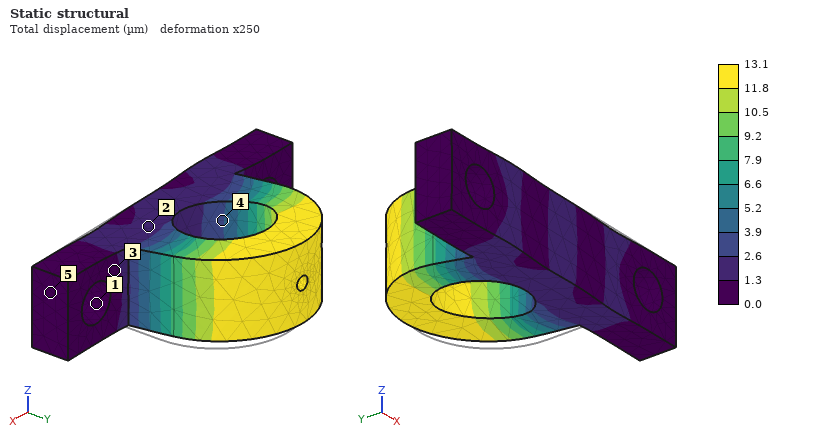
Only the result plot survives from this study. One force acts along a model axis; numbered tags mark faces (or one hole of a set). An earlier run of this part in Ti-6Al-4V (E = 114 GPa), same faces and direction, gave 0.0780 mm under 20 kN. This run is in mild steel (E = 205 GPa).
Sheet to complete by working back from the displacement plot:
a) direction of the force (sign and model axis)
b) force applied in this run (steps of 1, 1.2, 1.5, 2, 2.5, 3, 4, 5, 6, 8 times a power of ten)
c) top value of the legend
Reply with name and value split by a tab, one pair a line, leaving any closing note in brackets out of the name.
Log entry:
direction of the force	-X
force applied in this run	6 kN
top value of the legend	13.1 µm
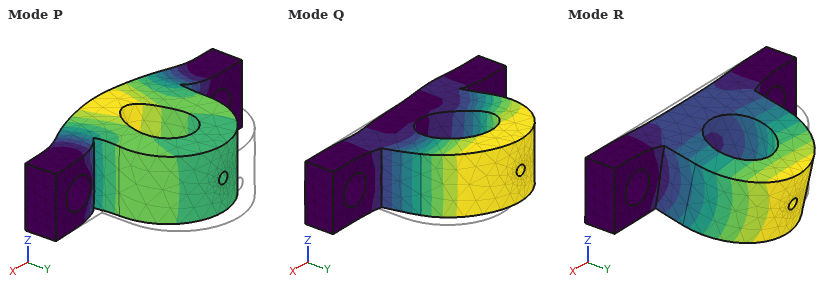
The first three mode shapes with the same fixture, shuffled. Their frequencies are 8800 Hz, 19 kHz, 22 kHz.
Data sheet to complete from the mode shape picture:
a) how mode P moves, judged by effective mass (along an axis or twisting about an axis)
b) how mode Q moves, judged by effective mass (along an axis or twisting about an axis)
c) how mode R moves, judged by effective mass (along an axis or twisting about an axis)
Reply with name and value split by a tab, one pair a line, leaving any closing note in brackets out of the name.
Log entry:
how mode P moves, judged by effective mass	along Y
how mode Q moves, judged by effective mass	along X
how mode R moves, judged by effective mass	along Z
